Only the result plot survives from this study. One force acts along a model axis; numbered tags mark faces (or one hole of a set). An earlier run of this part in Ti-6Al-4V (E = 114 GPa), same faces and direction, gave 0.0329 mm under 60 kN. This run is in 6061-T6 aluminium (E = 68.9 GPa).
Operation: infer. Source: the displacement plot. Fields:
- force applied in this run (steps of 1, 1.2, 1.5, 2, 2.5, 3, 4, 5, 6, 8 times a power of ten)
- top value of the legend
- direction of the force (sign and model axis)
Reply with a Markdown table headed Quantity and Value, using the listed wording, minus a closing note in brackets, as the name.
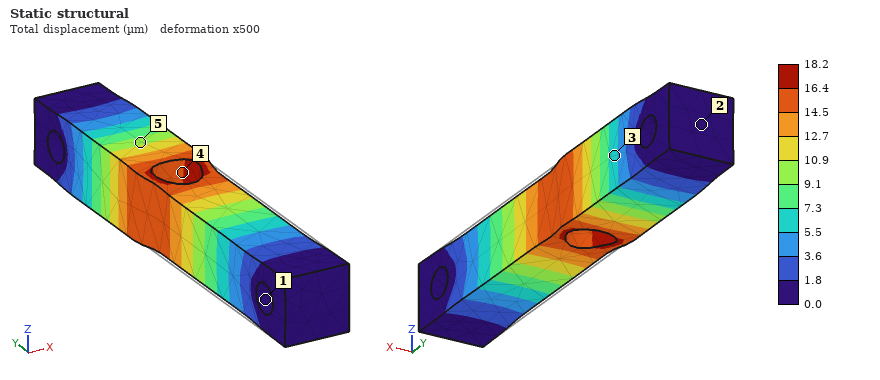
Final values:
| Quantity | Value |
|---|---|
| force applied in this run | 20 kN |
| top value of the legend | 18.2 µm |
| direction of the force | +Y |
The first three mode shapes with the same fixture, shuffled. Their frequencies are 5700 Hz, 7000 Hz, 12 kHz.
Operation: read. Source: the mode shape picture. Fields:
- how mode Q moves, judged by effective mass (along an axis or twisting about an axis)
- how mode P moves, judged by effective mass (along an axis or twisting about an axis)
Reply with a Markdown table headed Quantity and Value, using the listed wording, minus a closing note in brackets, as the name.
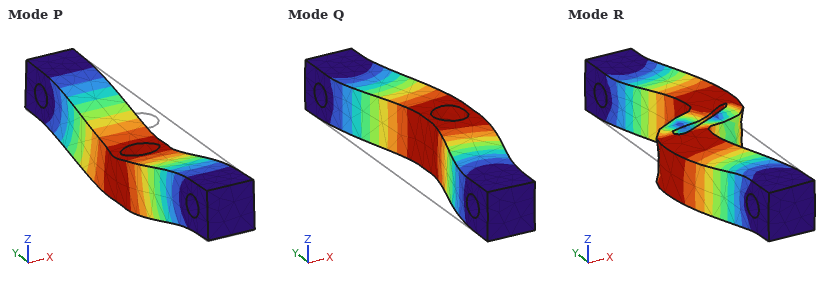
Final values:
| Quantity | Value |
|---|---|
| how mode Q moves, judged by effective mass | along X |
| how mode P moves, judged by effective mass | along Z |
